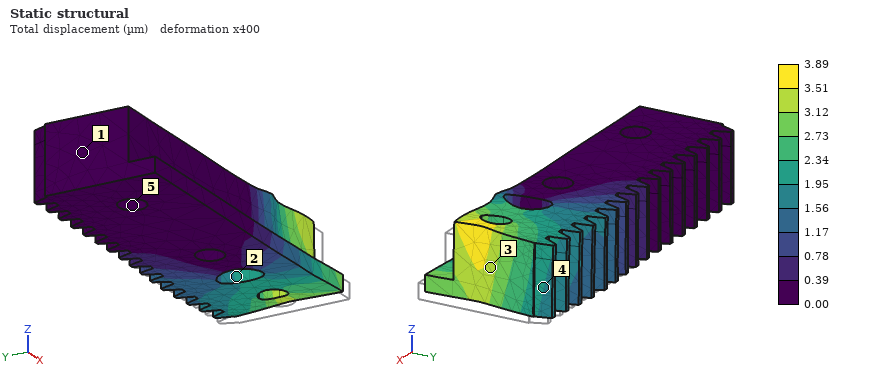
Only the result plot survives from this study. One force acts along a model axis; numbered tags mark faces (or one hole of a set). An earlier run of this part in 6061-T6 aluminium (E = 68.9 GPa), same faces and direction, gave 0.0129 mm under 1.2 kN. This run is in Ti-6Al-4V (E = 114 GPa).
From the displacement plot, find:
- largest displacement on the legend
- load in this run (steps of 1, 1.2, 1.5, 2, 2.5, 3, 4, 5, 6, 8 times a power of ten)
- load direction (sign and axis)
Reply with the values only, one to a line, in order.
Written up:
3.89 µm
600 N
-X
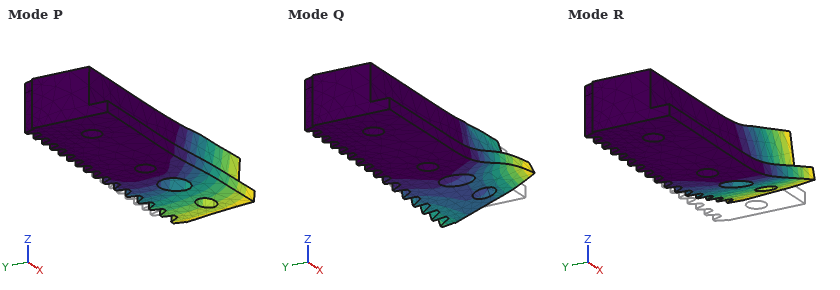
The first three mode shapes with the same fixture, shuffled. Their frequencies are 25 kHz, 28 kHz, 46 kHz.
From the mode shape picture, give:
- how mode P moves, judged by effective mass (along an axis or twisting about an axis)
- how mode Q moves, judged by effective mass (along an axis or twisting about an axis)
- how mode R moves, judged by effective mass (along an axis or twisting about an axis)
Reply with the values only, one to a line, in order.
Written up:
along Y
twisting about X
along Z
